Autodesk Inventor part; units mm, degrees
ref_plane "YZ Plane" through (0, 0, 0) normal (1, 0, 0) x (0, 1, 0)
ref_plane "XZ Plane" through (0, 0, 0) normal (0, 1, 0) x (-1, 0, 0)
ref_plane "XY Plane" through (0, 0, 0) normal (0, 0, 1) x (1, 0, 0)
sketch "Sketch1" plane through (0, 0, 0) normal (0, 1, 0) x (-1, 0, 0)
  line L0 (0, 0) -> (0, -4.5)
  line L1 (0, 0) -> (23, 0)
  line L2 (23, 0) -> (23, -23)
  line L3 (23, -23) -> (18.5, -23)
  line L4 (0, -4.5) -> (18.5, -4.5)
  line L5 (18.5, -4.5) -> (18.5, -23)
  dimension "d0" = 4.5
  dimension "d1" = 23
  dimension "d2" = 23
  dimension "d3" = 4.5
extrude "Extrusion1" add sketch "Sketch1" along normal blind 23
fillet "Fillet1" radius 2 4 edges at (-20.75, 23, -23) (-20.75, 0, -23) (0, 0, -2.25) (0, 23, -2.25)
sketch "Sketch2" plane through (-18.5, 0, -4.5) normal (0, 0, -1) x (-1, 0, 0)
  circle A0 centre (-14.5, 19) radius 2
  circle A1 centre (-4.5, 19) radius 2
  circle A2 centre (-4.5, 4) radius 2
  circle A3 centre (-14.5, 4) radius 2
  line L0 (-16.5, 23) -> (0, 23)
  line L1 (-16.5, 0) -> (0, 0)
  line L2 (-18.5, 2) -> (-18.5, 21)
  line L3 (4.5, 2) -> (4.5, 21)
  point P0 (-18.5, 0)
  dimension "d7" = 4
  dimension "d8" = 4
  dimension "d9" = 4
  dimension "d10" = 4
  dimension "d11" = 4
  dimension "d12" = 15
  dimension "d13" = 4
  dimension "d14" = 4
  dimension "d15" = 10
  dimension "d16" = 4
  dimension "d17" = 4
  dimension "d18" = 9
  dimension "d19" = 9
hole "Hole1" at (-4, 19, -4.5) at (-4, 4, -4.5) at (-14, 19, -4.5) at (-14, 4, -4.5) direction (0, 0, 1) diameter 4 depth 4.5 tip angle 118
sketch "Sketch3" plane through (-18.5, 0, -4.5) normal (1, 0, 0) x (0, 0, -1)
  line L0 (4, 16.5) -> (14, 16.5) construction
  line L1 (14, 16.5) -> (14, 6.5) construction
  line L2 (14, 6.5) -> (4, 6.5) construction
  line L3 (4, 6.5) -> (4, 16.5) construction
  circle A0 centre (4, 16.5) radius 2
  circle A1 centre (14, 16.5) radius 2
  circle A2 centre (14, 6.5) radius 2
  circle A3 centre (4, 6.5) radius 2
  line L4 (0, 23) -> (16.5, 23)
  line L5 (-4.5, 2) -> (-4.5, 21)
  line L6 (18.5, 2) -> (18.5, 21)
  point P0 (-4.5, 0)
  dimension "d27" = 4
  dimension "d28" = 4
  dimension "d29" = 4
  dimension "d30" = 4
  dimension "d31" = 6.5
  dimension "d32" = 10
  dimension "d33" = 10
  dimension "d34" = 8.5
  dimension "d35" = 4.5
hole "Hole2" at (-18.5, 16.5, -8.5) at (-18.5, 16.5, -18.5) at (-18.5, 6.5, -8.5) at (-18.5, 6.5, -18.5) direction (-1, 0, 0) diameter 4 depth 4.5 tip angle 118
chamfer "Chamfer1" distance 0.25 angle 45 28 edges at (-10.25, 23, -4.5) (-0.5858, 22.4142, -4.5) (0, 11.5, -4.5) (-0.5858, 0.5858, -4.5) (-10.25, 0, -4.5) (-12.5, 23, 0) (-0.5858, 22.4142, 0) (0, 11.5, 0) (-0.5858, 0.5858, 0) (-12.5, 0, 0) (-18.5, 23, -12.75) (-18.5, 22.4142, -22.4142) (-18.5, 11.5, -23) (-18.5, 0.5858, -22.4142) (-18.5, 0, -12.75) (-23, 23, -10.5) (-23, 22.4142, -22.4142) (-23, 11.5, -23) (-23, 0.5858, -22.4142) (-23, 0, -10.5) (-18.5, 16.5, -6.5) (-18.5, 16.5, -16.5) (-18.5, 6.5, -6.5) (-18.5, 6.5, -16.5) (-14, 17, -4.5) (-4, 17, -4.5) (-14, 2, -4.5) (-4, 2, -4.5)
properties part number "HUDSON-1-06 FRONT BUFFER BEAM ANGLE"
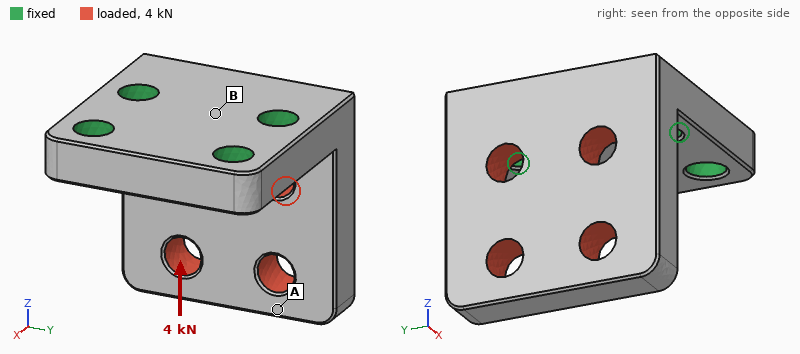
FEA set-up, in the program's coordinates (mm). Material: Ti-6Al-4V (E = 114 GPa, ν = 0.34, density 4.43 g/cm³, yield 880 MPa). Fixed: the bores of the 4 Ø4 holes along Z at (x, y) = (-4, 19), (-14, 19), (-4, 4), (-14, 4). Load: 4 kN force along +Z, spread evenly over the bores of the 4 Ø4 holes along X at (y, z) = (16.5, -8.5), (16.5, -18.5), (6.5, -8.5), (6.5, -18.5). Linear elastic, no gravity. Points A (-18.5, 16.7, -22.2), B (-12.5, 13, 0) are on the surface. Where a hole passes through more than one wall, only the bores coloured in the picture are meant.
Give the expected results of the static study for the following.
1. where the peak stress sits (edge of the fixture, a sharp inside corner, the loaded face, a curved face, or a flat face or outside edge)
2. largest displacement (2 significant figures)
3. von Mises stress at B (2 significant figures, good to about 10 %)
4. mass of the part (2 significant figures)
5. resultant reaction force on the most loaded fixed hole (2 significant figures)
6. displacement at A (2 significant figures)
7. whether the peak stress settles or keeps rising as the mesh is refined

edge of the fixture
97 µm
75 MPa
17 g
2.2 kN
88 µm
keeps rising
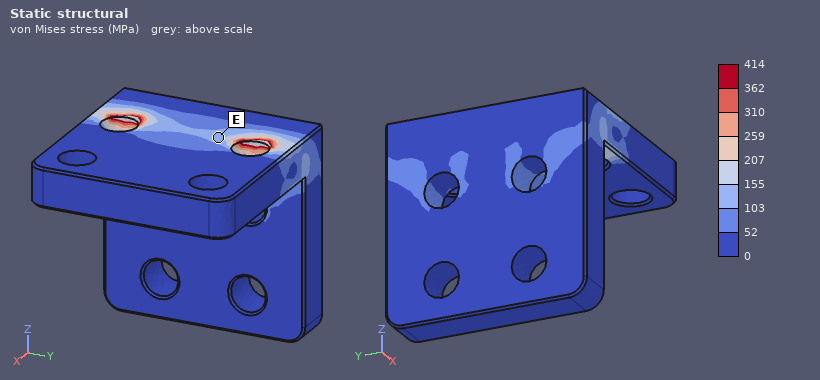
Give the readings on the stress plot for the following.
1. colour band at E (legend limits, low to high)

103 to 155 MPa
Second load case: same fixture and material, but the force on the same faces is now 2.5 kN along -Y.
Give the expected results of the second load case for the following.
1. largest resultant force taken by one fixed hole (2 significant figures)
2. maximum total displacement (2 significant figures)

2.2 kN
53 µm
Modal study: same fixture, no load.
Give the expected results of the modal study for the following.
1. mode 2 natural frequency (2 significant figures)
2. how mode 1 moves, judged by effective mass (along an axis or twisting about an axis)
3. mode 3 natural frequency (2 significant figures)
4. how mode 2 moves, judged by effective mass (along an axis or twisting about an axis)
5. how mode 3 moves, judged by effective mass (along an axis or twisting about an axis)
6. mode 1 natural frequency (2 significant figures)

13 kHz
along X
17 kHz
along Y
along Y
6200 Hz
